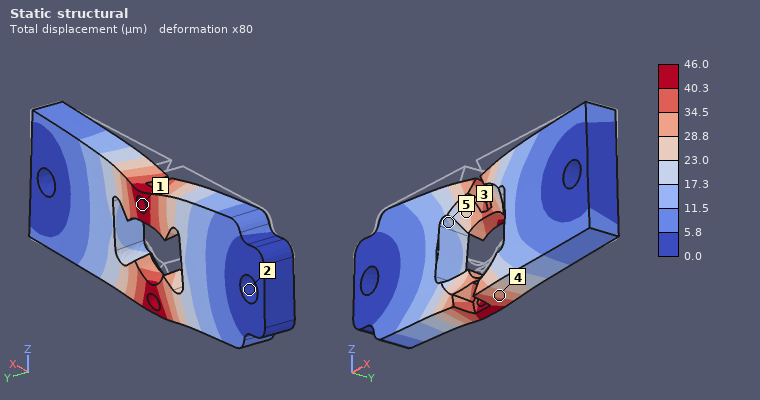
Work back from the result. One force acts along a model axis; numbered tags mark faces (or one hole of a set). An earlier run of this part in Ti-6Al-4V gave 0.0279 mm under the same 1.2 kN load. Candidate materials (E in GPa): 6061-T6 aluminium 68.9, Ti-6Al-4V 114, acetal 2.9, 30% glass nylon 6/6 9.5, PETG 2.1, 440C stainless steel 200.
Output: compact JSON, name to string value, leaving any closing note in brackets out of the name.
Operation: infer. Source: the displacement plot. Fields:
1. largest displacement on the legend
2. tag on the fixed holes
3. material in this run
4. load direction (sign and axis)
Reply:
{"largest displacement on the legend": "46.0 µm", "tag on the fixed holes": "2", "material in this run": "6061-T6 aluminium", "load direction": "-Z"}
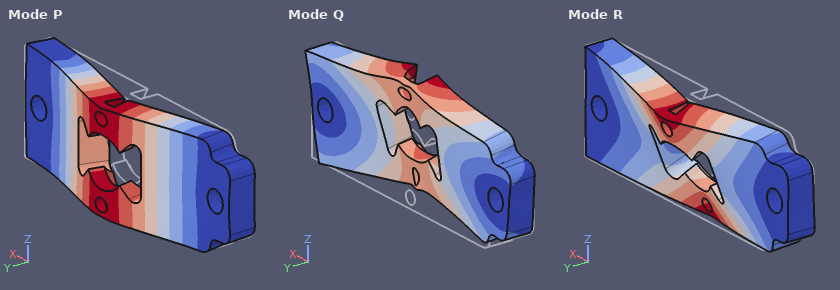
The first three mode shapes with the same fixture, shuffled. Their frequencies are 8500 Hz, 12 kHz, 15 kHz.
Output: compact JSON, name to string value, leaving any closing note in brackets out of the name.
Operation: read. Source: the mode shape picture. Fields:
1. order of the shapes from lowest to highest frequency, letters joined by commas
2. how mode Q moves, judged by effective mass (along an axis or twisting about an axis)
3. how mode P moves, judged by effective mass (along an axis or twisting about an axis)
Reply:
{"order of the shapes from lowest to highest frequency, letters joined by commas": "P, R, Q", "how mode Q moves, judged by effective mass": "along Z", "how mode P moves, judged by effective mass": "along Y"}
